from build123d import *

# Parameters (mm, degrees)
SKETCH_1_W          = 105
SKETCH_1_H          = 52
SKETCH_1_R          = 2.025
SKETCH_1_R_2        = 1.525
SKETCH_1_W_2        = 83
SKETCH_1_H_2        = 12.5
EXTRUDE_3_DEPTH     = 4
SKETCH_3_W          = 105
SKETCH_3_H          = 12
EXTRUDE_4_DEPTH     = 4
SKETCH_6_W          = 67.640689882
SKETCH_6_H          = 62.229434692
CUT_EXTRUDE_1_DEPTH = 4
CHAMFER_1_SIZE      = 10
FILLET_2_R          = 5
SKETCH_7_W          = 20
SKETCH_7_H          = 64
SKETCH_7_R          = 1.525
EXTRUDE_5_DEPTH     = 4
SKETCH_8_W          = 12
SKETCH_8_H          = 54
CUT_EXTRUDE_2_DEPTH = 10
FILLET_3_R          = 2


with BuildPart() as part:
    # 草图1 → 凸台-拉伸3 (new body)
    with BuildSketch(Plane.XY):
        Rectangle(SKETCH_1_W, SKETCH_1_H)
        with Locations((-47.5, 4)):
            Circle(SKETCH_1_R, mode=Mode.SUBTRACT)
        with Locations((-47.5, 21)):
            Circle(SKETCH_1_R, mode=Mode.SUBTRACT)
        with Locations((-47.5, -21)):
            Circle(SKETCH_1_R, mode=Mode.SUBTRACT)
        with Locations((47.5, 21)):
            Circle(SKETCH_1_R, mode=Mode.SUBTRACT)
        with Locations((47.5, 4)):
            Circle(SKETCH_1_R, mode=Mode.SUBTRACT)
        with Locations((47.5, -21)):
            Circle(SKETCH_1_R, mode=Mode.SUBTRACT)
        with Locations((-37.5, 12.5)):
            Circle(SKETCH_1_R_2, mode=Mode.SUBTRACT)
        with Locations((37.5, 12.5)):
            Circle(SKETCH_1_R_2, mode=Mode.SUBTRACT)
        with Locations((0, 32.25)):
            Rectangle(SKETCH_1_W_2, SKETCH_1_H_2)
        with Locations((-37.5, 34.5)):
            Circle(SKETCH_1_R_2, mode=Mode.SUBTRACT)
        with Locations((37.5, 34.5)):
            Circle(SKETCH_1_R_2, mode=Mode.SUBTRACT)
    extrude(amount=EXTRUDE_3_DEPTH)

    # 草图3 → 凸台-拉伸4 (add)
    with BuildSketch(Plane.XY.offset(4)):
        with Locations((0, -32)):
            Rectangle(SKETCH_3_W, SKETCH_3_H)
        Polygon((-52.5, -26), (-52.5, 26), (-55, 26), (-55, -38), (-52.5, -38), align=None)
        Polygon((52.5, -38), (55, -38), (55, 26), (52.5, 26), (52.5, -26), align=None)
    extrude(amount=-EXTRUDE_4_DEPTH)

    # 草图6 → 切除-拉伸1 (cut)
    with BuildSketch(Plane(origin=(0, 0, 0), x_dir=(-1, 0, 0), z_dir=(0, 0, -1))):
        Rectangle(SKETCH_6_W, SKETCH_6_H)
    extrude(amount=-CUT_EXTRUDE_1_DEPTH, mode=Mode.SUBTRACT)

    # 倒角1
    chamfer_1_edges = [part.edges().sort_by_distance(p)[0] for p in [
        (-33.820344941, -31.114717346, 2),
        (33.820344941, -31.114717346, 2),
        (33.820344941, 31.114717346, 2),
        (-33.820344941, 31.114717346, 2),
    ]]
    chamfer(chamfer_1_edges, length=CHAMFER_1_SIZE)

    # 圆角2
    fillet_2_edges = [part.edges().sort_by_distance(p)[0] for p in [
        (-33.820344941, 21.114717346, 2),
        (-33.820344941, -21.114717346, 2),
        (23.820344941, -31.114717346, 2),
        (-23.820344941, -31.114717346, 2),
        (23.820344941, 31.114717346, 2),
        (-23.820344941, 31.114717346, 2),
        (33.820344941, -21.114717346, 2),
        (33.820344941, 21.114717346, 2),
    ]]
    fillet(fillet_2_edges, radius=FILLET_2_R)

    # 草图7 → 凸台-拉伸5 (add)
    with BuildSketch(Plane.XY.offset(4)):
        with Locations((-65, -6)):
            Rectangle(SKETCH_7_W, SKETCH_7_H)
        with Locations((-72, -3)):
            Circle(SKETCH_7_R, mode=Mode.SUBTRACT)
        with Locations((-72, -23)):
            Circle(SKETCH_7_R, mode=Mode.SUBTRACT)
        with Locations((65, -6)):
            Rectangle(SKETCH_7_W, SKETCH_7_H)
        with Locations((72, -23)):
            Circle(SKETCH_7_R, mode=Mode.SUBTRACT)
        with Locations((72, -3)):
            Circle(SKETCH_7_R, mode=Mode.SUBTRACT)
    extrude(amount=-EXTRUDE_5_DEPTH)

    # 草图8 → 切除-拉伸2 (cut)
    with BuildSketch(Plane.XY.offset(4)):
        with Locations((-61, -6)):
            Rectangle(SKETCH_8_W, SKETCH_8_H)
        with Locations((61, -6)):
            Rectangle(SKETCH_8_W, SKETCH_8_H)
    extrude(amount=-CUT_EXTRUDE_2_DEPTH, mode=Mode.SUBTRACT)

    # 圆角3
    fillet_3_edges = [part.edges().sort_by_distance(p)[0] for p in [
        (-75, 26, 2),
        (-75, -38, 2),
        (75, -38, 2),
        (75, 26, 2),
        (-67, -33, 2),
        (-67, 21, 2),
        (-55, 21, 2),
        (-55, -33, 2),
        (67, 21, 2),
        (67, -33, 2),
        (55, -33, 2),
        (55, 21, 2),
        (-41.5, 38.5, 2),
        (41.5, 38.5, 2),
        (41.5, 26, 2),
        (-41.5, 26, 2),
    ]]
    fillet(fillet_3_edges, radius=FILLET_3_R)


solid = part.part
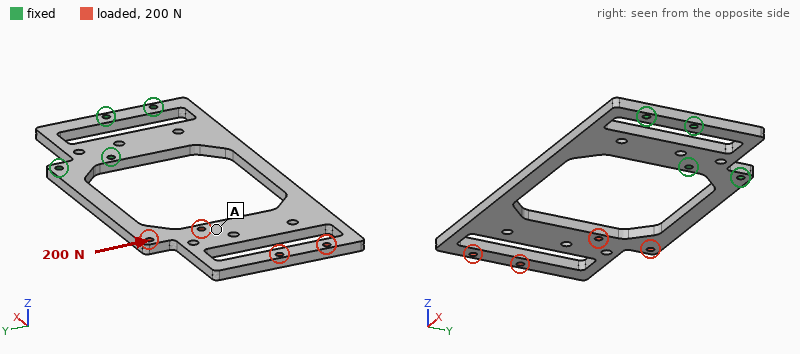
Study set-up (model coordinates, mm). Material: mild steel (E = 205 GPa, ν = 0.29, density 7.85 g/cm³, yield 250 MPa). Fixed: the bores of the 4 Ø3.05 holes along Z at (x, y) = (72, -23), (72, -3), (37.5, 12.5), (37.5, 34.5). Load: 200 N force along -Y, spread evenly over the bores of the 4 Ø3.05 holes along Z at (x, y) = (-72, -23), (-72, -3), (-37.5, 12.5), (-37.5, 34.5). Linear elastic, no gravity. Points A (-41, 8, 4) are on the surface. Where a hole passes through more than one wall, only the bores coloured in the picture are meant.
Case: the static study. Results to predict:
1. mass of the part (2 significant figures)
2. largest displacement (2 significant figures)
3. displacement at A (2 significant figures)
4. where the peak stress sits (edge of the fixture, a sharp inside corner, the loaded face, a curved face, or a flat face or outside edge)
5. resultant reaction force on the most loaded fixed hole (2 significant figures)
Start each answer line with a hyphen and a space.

- 160 g
- 89 µm
- 82 µm
- a curved face
- 380 N
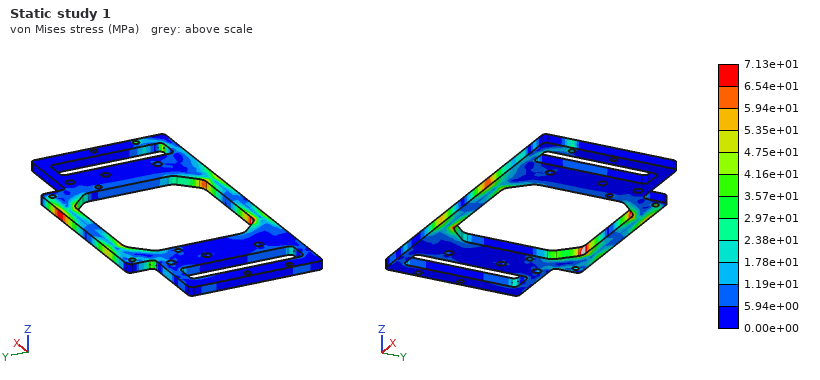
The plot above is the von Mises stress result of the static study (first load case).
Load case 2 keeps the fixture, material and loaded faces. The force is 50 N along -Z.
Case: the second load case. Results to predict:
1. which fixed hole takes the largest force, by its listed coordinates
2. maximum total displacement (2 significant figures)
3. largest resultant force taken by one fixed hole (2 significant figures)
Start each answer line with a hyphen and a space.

- (37.5, 34.5)
- 1.2 mm
- 43 N
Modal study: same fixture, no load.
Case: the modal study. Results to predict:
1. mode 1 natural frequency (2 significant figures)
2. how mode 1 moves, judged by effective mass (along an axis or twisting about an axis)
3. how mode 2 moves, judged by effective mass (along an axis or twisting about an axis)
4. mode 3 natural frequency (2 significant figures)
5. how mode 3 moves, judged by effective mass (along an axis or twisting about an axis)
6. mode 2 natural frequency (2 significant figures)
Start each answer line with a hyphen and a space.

- 150 Hz
- along Z
- twisting about X
- 890 Hz
- along Y
- 560 Hz
